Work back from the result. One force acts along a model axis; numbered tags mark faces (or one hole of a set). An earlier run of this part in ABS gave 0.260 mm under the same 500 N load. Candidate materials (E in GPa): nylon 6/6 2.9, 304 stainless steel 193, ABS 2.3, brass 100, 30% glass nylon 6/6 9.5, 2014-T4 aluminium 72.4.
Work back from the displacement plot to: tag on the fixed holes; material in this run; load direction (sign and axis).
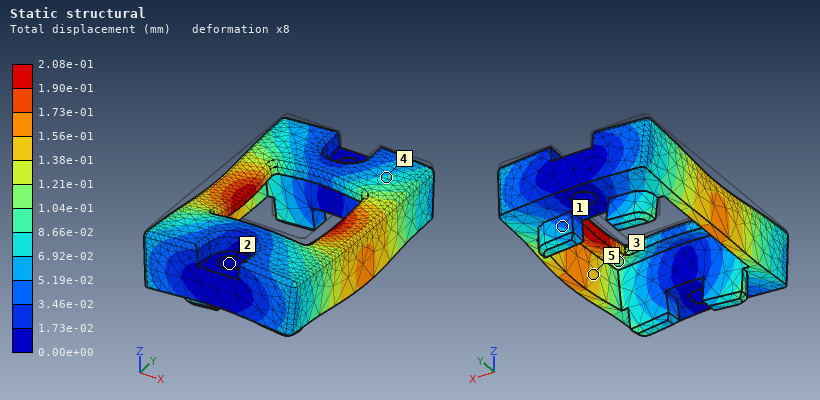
2
nylon 6/6
-Z
